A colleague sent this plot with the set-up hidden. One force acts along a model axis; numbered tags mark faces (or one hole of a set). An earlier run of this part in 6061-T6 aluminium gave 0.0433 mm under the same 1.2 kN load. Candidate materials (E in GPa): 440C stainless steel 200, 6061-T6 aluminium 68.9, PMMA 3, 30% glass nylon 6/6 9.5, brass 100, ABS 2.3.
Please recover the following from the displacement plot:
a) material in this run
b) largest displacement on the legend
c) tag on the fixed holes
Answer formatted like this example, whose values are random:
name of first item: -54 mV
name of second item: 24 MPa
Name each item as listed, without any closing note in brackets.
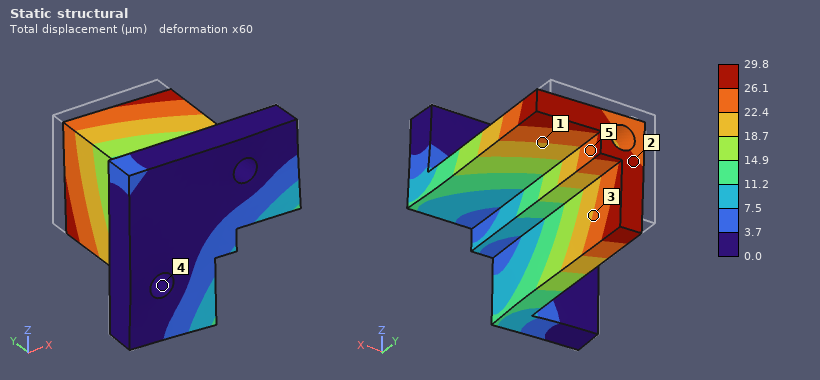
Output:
material in this run: brass
largest displacement on the legend: 29.8 µm
tag on the fixed holes: 4
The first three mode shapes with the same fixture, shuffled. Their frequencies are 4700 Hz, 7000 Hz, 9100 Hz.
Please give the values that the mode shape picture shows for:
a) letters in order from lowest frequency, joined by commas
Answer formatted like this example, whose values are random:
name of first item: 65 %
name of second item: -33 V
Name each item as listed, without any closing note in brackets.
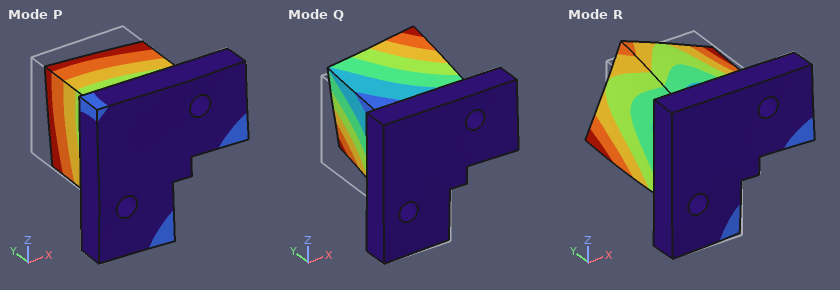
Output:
letters in order from lowest frequency, joined by commas: P, Q, R
